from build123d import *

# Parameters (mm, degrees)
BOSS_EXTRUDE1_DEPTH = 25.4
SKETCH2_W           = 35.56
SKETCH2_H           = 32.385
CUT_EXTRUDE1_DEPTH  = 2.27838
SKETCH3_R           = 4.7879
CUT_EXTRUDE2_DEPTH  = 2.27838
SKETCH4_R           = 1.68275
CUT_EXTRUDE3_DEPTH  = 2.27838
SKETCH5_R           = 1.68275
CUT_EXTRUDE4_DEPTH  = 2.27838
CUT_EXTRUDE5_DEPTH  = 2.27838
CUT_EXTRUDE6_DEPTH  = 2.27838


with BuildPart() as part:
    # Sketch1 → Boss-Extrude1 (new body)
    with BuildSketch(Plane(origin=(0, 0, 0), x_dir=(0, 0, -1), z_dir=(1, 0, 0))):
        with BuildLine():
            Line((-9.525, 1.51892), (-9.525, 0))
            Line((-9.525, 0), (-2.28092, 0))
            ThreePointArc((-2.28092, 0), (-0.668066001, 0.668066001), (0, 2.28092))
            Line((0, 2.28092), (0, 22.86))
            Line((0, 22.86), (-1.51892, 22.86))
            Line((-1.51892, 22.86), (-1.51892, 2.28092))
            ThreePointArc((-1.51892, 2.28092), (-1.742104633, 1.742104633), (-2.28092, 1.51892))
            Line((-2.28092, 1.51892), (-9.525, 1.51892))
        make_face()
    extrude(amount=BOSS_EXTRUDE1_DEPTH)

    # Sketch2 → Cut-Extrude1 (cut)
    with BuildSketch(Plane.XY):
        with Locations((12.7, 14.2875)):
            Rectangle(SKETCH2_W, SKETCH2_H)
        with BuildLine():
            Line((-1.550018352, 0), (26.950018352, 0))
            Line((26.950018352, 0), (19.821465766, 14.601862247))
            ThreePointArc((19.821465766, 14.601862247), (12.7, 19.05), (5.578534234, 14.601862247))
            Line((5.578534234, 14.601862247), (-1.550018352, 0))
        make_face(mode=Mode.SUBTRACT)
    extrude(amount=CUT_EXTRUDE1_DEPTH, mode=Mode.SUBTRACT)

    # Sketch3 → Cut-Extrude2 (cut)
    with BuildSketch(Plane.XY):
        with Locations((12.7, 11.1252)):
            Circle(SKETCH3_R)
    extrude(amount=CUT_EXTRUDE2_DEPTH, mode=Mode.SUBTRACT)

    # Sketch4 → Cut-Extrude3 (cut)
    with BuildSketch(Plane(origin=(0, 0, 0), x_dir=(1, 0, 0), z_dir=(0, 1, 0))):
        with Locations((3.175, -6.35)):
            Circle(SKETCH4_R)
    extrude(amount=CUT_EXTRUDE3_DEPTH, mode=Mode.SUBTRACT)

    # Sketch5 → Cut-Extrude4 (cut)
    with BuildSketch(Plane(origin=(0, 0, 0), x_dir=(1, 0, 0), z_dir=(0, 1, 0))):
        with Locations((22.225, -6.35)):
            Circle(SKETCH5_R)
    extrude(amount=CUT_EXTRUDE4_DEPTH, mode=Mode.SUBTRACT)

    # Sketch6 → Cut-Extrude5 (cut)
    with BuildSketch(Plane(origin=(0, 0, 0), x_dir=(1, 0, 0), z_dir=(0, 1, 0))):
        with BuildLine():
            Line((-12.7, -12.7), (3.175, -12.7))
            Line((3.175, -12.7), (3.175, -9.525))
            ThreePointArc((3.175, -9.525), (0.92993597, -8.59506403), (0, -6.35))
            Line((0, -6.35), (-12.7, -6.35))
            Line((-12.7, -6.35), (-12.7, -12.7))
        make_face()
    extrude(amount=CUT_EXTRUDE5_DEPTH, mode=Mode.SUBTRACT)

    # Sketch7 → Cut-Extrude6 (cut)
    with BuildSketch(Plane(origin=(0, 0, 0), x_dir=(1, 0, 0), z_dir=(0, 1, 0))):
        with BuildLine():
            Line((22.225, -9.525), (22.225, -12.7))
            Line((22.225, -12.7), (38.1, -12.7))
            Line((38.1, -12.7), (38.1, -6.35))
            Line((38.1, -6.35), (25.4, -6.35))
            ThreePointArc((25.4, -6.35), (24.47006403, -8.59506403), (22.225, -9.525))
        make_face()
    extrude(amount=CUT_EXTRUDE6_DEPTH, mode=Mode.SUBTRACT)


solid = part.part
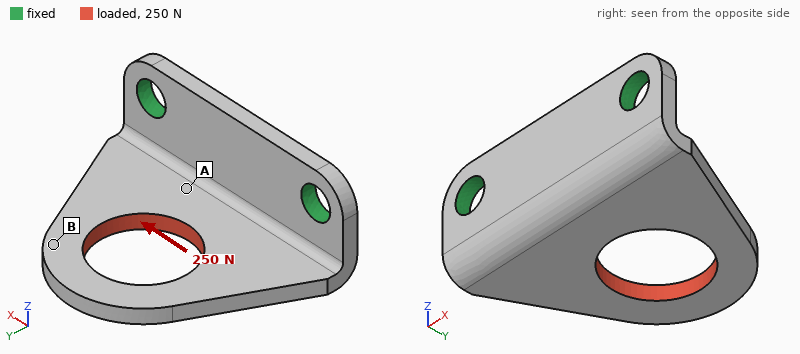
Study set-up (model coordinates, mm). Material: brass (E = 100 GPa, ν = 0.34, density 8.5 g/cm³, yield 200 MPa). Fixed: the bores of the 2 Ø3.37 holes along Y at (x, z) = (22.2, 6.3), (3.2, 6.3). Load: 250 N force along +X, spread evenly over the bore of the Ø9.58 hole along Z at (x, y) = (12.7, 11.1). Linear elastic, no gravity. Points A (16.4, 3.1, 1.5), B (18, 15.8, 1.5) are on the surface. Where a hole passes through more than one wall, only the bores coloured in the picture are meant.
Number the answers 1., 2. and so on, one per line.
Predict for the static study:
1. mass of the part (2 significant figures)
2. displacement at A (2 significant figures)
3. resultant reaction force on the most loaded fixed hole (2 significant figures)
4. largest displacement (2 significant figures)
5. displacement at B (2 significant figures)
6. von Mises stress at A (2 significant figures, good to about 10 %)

1. 5.7 g
2. 6.1 µm
3. 190 N
4. 35 µm
5. 33 µm
6. 41 MPa
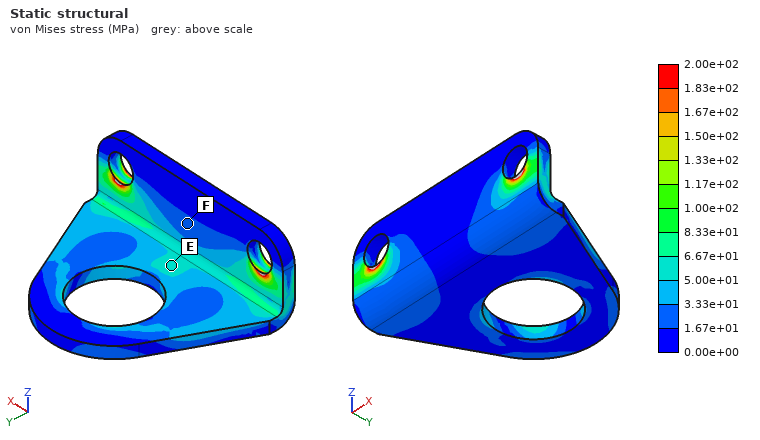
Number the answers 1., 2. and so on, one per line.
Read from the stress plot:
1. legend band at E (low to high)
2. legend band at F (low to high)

1. 5.00e+01 to 6.67e+01 MPa
2. 1.67e+01 to 3.33e+01 MPa
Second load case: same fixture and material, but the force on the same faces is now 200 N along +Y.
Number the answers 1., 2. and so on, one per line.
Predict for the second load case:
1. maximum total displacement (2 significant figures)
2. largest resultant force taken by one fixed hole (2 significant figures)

1. 63 µm
2. 100 N
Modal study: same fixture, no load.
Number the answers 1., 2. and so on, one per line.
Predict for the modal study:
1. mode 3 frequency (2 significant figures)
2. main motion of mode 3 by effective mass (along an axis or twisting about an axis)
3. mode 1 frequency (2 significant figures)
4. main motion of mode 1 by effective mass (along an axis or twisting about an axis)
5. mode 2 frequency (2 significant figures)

1. 10000 Hz
2. along Y
3. 2800 Hz
4. along Z
5. 7000 Hz
